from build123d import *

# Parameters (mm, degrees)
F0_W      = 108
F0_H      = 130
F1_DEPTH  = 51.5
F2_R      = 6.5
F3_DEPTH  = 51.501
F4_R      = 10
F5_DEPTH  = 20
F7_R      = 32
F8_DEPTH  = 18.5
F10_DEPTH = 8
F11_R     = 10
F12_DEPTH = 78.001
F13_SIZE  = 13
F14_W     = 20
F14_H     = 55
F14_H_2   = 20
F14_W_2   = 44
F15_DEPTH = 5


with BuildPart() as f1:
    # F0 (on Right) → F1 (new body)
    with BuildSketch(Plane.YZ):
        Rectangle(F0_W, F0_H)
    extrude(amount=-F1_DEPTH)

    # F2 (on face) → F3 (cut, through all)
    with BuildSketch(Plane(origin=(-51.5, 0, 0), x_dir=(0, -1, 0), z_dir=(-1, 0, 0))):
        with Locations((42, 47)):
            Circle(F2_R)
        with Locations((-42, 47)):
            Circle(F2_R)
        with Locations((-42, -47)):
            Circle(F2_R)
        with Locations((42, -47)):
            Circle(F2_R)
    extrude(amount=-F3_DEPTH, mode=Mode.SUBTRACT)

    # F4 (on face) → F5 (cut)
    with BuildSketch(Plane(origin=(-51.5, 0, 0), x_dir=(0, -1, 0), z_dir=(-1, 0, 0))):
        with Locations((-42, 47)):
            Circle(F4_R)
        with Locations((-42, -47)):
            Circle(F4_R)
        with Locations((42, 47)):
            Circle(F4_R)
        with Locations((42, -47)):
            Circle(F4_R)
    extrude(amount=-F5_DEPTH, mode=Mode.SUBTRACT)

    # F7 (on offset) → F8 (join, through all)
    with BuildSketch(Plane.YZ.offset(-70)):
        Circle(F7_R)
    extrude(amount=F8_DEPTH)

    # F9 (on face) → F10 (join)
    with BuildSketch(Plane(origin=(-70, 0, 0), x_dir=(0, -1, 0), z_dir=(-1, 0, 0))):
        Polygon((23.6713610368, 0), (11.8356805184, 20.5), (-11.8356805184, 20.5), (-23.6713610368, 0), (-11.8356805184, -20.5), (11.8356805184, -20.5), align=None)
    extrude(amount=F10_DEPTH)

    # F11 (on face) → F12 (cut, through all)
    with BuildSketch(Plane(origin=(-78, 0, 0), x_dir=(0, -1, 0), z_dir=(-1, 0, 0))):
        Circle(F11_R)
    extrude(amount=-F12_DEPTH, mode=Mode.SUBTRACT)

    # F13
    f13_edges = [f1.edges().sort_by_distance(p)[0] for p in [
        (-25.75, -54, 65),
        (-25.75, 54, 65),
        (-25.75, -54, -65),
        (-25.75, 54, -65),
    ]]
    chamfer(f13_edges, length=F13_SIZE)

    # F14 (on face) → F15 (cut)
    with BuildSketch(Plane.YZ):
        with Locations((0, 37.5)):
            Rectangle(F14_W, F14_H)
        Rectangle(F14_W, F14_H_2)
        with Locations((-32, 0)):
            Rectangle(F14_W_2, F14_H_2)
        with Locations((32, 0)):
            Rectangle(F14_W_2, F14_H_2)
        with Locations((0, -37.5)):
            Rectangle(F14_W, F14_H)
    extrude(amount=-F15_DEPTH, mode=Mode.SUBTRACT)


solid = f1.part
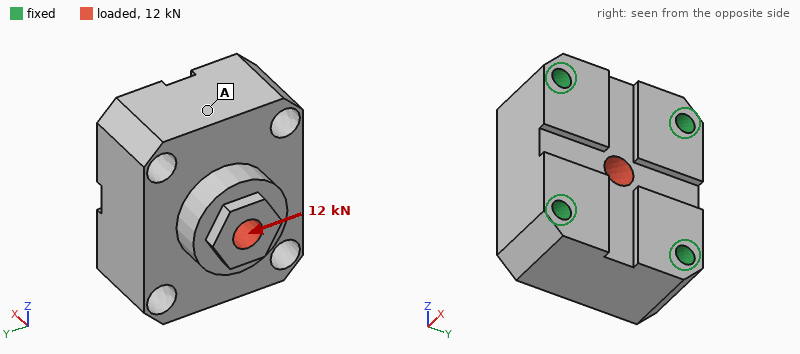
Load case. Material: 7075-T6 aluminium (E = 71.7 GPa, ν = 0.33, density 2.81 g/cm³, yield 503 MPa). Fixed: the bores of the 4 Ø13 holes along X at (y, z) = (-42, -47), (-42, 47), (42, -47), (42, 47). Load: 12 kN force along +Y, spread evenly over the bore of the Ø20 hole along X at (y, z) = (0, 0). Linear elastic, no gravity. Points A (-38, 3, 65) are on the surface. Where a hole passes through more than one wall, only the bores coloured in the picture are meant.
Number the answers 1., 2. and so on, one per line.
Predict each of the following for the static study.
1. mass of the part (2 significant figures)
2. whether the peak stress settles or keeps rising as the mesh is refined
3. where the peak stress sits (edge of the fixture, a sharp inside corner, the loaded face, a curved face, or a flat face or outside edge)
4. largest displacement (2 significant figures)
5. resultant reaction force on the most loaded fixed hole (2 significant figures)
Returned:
1. 1.9 kg
2. keeps rising
3. edge of the fixture
4. 6.2 µm
5. 3.8 kN
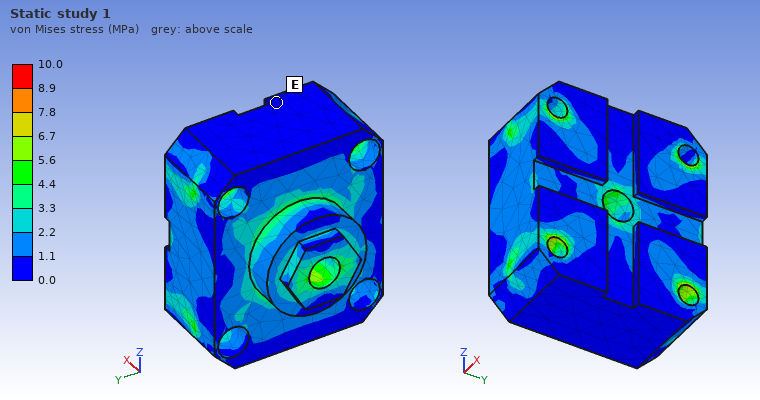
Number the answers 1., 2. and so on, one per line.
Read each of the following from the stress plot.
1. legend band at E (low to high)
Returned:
1. 0.0 to 1.1 MPa
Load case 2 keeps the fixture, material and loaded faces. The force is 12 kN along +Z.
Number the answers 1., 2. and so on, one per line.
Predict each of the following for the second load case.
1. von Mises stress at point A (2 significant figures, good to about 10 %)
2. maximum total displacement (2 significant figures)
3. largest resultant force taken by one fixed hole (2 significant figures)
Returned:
1. 1.2 MPa
2. 5.4 µm
3. 3.5 kN
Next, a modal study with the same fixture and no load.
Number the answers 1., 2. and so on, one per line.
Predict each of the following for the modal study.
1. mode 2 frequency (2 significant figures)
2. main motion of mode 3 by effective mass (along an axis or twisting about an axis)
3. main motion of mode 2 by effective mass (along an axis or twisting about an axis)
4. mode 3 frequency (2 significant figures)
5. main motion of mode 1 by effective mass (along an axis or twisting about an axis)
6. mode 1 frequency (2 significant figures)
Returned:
1. 10 kHz
2. along Z
3. along Y
4. 11 kHz
5. along X
6. 9600 Hz
